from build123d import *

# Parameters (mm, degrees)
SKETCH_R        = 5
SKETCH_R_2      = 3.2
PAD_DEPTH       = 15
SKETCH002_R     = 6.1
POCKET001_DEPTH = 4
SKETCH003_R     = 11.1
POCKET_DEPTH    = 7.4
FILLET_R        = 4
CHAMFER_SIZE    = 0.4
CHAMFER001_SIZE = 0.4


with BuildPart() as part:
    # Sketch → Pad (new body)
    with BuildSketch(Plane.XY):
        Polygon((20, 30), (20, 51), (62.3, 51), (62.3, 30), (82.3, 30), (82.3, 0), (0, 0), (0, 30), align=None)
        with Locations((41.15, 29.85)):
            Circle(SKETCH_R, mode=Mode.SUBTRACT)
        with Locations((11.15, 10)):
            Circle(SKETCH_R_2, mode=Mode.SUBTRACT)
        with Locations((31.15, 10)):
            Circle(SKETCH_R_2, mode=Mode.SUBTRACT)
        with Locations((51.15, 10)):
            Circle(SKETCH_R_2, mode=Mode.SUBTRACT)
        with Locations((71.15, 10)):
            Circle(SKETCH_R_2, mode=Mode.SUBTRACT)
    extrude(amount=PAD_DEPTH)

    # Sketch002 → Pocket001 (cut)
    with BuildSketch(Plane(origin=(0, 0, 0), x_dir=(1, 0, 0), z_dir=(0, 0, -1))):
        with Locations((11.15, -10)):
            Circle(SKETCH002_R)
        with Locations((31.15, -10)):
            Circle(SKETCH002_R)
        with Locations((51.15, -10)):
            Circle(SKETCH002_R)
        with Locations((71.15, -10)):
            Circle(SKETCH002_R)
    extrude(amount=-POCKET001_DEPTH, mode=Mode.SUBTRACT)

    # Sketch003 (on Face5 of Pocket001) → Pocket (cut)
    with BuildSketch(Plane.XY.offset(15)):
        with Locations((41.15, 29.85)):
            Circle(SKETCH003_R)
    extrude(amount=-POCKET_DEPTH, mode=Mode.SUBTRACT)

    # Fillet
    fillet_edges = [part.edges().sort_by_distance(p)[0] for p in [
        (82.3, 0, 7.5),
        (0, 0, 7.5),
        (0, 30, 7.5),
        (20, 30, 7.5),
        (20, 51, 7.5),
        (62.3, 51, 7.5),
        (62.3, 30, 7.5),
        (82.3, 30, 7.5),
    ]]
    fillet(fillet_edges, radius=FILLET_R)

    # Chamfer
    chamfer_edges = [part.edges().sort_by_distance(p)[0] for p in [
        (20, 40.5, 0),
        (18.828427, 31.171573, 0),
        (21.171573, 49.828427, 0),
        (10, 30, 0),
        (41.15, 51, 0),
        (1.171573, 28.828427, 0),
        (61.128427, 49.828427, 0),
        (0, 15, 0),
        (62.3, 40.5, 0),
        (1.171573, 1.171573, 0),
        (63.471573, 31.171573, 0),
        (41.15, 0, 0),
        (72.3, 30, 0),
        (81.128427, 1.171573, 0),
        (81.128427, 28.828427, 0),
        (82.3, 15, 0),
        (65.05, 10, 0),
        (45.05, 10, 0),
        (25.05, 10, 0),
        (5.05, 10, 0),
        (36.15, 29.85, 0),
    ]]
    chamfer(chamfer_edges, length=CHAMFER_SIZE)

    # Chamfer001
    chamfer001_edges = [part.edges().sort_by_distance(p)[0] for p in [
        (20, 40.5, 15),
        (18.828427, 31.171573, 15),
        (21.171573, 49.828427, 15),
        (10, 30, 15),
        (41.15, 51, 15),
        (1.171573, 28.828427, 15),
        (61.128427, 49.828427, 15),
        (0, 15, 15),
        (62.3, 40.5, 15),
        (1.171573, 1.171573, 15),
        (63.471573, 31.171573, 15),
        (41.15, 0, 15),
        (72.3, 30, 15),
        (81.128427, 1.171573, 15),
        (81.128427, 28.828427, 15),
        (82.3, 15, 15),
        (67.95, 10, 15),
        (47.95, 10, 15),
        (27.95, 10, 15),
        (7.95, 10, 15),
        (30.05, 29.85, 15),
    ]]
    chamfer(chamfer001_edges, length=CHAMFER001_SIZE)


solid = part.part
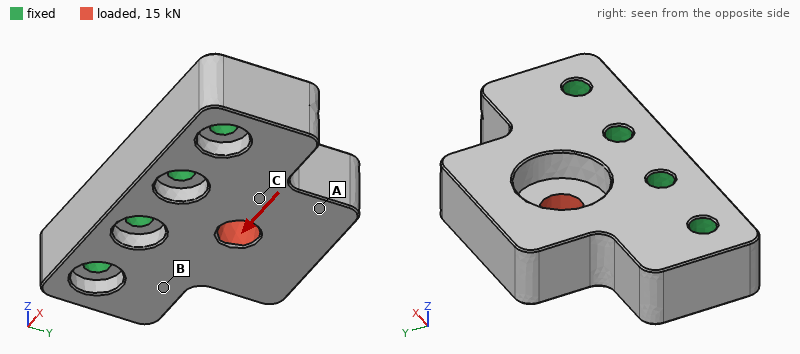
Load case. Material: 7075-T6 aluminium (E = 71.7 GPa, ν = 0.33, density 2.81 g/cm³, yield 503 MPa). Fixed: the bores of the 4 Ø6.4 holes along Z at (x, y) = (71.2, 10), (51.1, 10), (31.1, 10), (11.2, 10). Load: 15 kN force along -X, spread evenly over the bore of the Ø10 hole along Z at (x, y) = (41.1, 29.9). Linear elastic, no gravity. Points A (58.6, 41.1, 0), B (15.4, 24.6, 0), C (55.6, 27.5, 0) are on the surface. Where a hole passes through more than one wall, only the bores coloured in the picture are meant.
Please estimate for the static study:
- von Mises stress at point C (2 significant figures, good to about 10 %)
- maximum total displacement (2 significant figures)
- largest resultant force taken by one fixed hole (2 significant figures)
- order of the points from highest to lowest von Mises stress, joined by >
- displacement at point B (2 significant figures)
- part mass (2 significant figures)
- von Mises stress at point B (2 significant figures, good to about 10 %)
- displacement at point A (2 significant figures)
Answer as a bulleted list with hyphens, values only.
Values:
- 53 MPa
- 28 µm
- 5.6 kN
- C > B > A
- 9.2 µm
- 120 g
- 26 MPa
- 23 µm
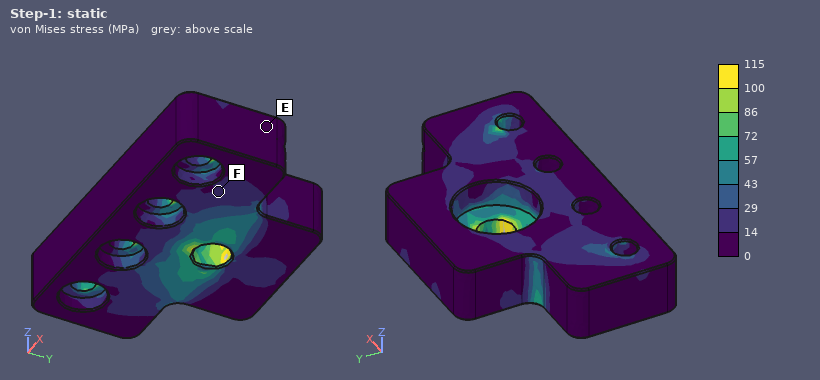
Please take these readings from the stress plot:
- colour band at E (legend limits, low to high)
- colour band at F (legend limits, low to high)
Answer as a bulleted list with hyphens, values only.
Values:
- 0 to 14 MPa
- 14 to 29 MPa
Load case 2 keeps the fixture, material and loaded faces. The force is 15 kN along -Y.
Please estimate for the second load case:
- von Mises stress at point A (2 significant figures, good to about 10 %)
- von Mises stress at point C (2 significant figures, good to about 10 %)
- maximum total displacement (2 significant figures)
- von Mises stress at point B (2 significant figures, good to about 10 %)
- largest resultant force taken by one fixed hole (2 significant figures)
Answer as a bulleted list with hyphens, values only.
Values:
- 16 MPa
- 29 MPa
- 51 µm
- 23 MPa
- 5.7 kN
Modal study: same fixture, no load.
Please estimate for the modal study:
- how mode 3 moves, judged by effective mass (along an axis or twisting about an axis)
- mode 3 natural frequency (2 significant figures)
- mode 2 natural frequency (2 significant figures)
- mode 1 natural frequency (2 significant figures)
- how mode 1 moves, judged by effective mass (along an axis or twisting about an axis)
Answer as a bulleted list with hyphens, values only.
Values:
- along X
- 17 kHz
- 13 kHz
- 6400 Hz
- along Z
